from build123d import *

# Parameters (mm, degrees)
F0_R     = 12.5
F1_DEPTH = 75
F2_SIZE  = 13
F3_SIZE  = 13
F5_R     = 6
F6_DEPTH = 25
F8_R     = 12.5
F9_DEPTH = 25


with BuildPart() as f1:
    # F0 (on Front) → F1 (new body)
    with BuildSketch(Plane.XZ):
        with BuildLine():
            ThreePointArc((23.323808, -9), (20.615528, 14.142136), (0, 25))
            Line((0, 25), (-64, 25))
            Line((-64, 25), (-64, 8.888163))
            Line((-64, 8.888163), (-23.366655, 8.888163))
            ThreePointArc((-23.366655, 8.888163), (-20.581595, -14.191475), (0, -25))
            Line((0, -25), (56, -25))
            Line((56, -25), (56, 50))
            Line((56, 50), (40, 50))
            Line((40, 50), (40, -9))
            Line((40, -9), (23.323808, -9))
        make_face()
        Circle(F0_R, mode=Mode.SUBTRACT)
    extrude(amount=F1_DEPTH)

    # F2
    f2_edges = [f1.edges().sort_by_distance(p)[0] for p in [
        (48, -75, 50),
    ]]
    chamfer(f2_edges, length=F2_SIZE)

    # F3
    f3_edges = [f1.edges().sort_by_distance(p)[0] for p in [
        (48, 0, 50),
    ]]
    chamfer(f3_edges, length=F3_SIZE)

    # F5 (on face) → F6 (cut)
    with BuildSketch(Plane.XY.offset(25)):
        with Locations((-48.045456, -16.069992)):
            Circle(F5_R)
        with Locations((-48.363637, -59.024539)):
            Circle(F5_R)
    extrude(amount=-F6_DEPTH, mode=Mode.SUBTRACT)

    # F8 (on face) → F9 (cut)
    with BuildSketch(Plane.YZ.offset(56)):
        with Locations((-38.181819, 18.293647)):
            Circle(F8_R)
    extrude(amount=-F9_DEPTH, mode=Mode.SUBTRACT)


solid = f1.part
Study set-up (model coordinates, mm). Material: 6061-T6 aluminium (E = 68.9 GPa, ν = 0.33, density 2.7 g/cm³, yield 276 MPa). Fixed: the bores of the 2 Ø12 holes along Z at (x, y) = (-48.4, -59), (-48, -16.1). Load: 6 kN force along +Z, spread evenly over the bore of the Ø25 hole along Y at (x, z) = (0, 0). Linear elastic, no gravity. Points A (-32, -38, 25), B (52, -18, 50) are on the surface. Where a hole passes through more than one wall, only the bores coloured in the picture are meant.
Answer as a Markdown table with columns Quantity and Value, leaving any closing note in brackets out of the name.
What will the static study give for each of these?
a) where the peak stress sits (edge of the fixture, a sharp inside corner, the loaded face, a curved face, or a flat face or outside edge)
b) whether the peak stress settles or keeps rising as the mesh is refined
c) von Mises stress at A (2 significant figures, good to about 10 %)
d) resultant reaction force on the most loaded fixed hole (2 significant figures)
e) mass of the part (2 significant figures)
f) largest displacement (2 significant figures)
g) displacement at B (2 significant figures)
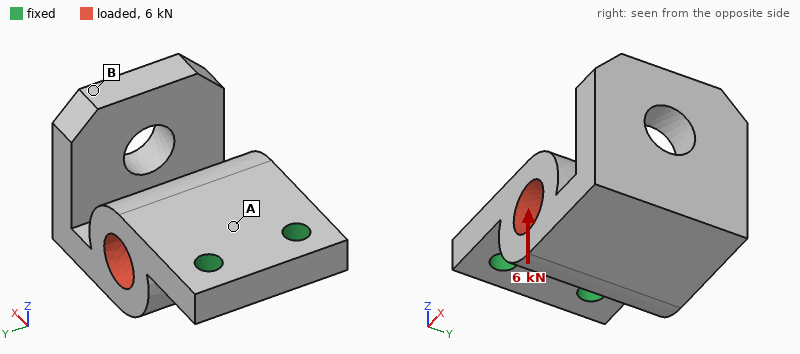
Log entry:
| Quantity | Value |
|---|---|
| where the peak stress sits | edge of the fixture |
| whether the peak stress settles or keeps rising as the mesh is refined | keeps rising |
| von Mises stress at A | 45 MPa |
| resultant reaction force on the most loaded fixed hole | 3.0 kN |
| mass of the part | 730 g |
| largest displacement | 0.33 mm |
| displacement at B | 0.31 mm |
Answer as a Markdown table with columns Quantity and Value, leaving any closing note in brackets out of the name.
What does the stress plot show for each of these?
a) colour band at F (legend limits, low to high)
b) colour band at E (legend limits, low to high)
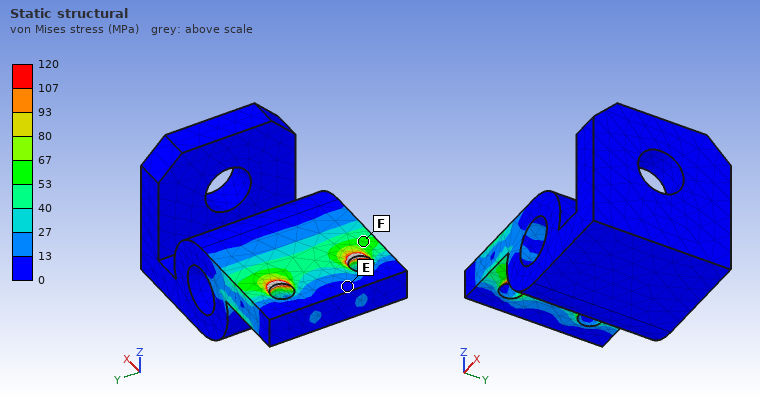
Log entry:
| Quantity | Value |
|---|---|
| colour band at F | 53 to 67 MPa |
| colour band at E | 0 to 13 MPa |
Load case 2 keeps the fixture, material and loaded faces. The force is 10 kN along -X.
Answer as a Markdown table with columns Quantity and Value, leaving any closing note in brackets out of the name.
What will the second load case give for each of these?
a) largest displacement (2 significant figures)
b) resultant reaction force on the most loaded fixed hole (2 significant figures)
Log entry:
| Quantity | Value |
|---|---|
| largest displacement | 0.29 mm |
| resultant reaction force on the most loaded fixed hole | 5.1 kN |
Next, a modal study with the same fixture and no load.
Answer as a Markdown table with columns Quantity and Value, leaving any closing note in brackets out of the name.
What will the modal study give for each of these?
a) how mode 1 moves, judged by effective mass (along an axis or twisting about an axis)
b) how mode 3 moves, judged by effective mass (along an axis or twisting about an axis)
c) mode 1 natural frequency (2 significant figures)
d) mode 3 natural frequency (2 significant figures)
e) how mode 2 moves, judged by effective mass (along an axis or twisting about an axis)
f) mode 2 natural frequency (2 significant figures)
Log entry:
| Quantity | Value |
|---|---|
| how mode 1 moves, judged by effective mass | along Z |
| how mode 3 moves, judged by effective mass | along Y |
| mode 1 natural frequency | 760 Hz |
| mode 3 natural frequency | 2000 Hz |
| how mode 2 moves, judged by effective mass | along X |
| mode 2 natural frequency | 1900 Hz |
